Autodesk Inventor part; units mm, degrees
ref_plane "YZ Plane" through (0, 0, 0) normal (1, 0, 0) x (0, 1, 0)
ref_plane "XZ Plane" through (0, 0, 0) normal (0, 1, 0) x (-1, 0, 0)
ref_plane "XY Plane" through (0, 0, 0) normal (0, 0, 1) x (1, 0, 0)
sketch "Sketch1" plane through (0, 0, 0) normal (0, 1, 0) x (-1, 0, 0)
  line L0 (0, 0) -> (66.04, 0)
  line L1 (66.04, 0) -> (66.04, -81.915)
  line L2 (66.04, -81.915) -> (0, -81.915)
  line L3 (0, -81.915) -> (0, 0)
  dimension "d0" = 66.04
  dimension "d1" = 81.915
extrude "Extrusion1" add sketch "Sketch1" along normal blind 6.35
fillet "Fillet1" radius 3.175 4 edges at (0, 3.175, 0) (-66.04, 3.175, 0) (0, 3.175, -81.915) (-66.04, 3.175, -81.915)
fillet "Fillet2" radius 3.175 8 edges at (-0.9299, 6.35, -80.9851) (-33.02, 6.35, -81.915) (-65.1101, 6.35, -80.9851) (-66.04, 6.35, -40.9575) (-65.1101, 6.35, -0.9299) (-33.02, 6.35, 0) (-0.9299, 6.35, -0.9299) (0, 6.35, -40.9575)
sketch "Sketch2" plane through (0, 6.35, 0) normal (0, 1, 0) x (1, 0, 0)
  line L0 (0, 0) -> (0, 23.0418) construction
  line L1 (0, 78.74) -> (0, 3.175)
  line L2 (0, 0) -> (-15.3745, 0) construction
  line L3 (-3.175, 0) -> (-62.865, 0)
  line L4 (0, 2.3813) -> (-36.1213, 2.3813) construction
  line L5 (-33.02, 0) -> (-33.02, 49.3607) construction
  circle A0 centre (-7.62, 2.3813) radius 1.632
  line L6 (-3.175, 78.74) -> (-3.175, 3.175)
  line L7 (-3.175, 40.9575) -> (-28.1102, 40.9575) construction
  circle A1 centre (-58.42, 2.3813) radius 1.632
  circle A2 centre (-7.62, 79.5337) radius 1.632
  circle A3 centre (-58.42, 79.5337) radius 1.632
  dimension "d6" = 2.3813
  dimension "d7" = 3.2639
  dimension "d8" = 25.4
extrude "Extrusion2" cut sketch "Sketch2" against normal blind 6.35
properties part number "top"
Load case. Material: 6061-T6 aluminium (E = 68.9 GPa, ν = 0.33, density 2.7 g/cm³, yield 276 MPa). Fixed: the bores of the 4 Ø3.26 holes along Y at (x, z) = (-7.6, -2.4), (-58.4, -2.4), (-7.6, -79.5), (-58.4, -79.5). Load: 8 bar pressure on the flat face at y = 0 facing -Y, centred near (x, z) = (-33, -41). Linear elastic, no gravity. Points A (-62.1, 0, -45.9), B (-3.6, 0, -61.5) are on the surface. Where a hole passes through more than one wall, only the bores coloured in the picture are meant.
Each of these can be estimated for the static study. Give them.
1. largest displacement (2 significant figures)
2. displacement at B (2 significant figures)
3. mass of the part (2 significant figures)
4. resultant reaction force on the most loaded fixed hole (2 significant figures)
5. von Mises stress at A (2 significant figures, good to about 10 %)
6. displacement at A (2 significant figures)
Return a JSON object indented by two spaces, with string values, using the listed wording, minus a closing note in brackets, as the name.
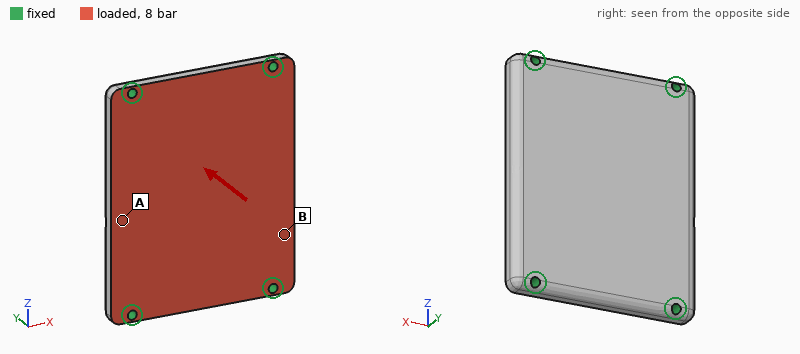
{
  "largest displacement": "97 µm",
  "displacement at B": "50 µm",
  "mass of the part": "90 g",
  "resultant reaction force on the most loaded fixed hole": "1.1 kN",
  "von Mises stress at A": "41 MPa",
  "displacement at A": "86 µm"
}
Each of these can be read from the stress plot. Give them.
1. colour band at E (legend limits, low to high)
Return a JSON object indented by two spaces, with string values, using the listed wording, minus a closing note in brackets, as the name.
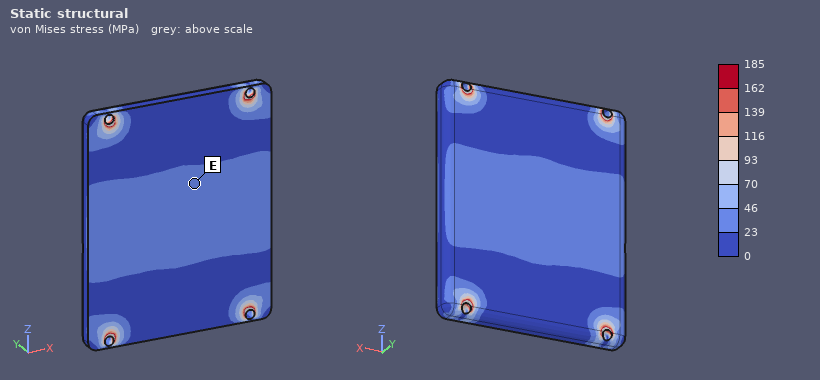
{
  "colour band at E": "23 to 46 MPa"
}
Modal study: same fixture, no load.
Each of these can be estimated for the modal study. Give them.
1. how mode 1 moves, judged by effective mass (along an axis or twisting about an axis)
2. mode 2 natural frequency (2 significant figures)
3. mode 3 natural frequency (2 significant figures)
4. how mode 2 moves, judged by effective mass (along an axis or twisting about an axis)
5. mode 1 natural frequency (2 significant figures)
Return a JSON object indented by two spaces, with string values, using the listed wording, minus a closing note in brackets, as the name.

{
  "how mode 1 moves, judged by effective mass": "along Y",
  "mode 2 natural frequency": "6200 Hz",
  "mode 3 natural frequency": "9700 Hz",
  "how mode 2 moves, judged by effective mass": "twisting about Z",
  "mode 1 natural frequency": "4000 Hz"
}
